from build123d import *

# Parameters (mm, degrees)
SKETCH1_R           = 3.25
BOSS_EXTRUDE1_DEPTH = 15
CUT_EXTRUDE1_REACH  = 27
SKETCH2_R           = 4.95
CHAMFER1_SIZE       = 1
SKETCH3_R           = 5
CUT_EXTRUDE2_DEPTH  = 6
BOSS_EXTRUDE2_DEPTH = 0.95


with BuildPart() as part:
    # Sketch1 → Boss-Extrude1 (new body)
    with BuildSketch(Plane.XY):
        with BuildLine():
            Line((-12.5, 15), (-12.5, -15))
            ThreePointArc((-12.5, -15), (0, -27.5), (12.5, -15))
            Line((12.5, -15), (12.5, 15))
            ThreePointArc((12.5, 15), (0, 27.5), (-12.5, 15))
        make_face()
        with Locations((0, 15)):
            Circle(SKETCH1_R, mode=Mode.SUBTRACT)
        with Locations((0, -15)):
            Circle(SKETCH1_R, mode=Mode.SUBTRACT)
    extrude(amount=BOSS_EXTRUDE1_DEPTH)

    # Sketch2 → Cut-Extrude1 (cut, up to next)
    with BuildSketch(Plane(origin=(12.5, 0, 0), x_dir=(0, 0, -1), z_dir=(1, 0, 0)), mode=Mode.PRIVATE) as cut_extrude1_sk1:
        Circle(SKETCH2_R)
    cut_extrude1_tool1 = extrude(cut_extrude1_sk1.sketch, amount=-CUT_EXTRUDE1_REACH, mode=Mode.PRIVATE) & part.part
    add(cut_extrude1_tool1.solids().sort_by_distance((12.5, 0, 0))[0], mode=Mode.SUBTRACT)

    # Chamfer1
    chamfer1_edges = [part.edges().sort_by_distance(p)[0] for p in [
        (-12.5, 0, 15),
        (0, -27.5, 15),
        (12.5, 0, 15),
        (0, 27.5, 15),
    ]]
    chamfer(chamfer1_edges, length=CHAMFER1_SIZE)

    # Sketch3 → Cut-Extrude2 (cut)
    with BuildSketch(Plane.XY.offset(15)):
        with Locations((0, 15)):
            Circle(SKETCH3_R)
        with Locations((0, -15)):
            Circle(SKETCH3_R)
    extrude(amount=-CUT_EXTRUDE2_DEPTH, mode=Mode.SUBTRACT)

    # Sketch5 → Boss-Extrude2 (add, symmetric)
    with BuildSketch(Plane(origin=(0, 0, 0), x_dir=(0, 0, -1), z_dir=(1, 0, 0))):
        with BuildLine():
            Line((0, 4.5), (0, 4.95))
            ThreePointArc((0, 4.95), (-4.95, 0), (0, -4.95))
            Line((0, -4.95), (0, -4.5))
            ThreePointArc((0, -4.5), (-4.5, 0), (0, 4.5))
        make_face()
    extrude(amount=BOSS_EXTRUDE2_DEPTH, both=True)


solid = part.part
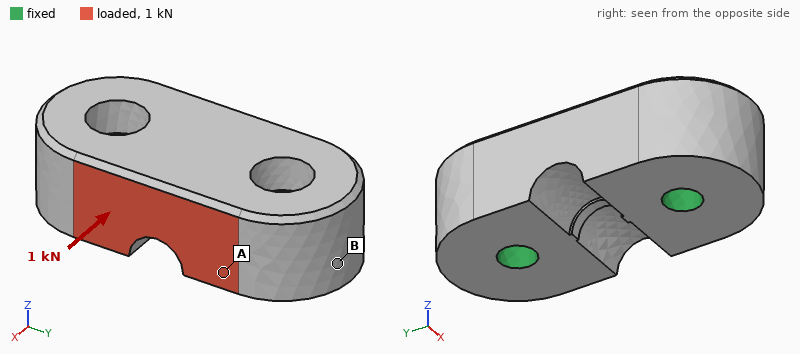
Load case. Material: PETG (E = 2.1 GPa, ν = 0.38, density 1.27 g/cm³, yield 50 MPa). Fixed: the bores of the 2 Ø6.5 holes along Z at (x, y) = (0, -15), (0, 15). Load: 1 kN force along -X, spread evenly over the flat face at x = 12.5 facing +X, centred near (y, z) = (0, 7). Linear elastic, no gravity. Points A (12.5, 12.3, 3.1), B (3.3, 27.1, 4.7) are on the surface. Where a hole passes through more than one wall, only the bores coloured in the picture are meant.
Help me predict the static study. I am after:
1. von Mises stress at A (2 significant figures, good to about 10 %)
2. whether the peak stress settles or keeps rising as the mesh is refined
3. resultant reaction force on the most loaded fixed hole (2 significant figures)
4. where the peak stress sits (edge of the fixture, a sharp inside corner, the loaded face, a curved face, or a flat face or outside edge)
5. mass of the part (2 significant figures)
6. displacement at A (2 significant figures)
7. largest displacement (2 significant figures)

2.4 MPa
keeps rising
510 N
edge of the fixture
20 g
25 µm
57 µm
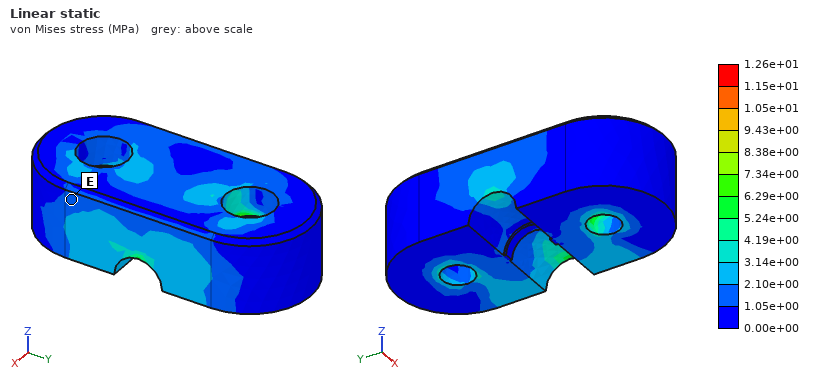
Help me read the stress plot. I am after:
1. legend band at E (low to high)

1.05e+00 to 2.10e+00 MPa
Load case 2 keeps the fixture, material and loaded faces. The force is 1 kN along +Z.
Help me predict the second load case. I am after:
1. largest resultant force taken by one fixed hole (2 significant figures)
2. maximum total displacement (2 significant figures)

540 N
0.19 mm
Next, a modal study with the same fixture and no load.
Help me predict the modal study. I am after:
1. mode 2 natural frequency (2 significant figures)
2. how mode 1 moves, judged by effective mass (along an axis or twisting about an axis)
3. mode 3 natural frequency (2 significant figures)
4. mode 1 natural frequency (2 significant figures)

8000 Hz
along X
8200 Hz
5800 Hz
